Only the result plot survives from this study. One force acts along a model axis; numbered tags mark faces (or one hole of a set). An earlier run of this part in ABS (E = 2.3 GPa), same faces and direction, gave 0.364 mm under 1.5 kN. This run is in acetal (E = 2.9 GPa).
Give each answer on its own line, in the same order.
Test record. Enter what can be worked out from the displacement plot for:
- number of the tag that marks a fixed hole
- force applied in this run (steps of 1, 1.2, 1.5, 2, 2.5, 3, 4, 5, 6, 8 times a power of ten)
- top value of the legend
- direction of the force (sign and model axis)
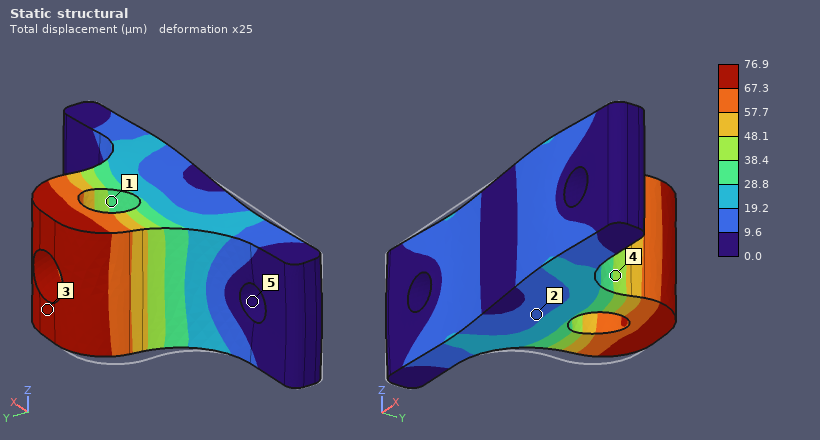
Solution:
5
400 N
76.9 µm
+X
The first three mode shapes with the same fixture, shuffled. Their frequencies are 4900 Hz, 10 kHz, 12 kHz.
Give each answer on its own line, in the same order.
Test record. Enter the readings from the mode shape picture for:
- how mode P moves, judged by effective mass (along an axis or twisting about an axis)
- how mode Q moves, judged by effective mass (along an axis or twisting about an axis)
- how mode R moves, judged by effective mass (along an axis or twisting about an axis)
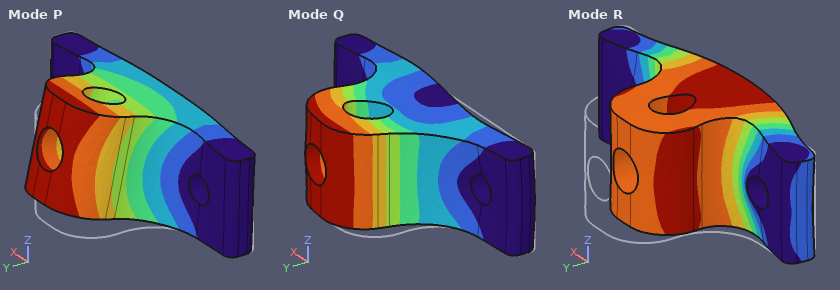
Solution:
along Z
along X
along Y
